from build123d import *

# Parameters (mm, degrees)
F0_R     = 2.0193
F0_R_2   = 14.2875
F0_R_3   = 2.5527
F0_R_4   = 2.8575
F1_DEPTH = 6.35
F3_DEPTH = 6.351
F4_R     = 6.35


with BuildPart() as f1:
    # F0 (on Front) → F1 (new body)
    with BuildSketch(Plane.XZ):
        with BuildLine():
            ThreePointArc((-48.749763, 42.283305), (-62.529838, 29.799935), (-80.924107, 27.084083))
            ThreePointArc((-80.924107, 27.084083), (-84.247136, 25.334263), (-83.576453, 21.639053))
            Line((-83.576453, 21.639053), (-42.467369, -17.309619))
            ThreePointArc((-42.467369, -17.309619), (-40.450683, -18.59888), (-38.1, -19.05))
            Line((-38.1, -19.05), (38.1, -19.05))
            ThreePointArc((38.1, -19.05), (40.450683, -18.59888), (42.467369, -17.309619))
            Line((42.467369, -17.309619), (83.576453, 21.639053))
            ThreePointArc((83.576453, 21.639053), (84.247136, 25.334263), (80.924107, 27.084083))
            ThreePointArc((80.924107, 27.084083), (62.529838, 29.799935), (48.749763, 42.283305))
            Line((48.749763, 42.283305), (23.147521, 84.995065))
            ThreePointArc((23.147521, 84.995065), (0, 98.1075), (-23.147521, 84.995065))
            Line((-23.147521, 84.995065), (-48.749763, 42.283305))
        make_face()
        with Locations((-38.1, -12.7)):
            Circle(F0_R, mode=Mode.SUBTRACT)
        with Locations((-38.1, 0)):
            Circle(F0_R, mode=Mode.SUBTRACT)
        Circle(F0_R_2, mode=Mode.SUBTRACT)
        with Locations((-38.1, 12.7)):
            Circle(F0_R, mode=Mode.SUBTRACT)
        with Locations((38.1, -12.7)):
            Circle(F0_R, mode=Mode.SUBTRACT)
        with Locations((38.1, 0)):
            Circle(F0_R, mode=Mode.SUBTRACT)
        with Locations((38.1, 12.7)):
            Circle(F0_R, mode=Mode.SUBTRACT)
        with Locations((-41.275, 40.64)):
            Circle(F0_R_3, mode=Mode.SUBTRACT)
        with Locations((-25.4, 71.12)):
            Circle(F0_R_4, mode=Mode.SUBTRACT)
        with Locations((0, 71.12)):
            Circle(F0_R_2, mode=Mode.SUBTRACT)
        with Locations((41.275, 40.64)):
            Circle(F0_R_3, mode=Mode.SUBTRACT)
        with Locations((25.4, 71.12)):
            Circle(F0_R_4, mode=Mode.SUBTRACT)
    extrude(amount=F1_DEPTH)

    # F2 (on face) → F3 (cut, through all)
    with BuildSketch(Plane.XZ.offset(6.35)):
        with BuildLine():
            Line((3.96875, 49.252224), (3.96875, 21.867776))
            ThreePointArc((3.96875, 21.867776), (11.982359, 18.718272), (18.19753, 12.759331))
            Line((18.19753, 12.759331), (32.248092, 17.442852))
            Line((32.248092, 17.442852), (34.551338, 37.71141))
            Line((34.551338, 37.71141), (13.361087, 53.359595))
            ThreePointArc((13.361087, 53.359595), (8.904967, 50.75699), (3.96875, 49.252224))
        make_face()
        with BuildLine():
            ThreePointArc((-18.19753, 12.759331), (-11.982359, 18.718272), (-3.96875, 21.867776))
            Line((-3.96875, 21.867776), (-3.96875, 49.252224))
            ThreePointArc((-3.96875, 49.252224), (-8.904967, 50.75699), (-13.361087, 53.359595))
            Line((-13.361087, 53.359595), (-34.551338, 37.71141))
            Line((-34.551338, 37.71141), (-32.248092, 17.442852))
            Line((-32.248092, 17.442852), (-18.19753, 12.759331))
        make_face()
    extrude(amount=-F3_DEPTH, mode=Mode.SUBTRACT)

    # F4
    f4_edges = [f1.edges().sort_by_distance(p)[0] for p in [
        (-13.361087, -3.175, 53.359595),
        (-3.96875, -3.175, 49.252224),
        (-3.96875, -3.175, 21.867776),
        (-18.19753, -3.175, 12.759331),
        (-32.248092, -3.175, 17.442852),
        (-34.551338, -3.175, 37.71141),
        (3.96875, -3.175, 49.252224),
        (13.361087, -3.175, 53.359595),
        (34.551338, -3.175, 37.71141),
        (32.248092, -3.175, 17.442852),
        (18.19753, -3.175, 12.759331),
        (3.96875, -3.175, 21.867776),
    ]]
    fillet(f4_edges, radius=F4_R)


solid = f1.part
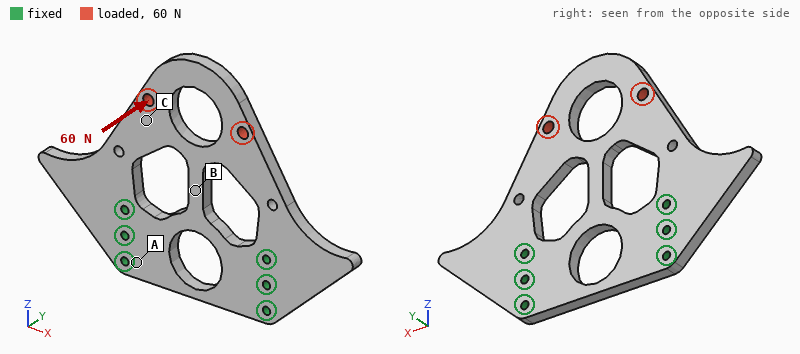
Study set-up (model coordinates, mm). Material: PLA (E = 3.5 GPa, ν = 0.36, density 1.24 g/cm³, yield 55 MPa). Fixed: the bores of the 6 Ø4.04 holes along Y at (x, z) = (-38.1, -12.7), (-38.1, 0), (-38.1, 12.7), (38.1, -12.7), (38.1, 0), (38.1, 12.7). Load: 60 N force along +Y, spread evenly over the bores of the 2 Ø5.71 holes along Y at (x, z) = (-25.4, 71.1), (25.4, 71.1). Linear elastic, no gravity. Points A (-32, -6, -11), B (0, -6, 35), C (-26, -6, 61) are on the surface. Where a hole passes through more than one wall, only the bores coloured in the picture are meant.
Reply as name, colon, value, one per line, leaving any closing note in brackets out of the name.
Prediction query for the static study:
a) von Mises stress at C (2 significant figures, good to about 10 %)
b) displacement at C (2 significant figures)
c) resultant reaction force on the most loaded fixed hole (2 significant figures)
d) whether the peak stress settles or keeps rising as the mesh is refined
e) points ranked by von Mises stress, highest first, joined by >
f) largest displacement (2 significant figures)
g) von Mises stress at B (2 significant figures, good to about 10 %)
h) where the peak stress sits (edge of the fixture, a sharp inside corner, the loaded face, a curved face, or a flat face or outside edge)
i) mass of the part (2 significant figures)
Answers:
von Mises stress at C: 2.6 MPa
displacement at C: 0.88 mm
resultant reaction force on the most loaded fixed hole: 87 N
whether the peak stress settles or keeps rising as the mesh is refined: keeps rising
points ranked by von Mises stress, highest first, joined by >: B > C > A
largest displacement: 2.1 mm
von Mises stress at B: 6.3 MPa
where the peak stress sits: edge of the fixture
mass of the part: 63 g
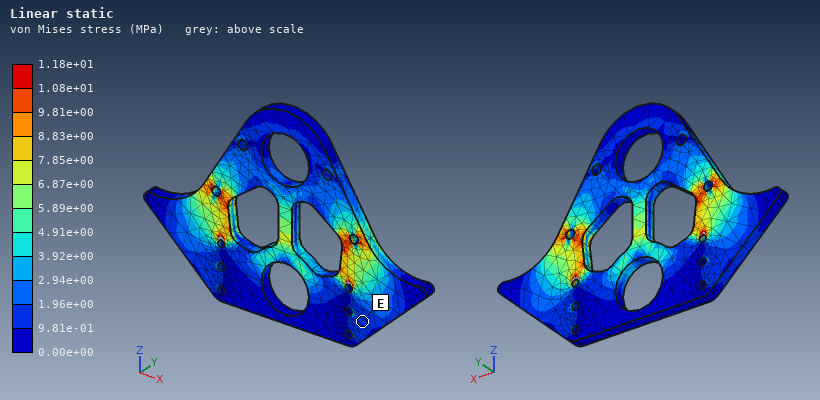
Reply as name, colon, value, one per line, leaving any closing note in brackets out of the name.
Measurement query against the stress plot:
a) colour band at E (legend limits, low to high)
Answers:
colour band at E: 9.81e-01 to 1.96e+00 MPa
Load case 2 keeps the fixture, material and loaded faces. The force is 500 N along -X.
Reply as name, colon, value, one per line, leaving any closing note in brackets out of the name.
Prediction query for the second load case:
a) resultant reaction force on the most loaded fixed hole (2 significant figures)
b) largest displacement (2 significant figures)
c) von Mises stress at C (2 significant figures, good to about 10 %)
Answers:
resultant reaction force on the most loaded fixed hole: 400 N
largest displacement: 0.23 mm
von Mises stress at C: 2.0 MPa
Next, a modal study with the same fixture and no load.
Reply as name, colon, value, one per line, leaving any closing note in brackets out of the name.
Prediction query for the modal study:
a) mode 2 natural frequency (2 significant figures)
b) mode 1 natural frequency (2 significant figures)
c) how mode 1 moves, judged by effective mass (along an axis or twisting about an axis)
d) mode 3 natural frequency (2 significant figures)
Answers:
mode 2 natural frequency: 810 Hz
mode 1 natural frequency: 260 Hz
how mode 1 moves, judged by effective mass: along Y
mode 3 natural frequency: 1200 Hz
